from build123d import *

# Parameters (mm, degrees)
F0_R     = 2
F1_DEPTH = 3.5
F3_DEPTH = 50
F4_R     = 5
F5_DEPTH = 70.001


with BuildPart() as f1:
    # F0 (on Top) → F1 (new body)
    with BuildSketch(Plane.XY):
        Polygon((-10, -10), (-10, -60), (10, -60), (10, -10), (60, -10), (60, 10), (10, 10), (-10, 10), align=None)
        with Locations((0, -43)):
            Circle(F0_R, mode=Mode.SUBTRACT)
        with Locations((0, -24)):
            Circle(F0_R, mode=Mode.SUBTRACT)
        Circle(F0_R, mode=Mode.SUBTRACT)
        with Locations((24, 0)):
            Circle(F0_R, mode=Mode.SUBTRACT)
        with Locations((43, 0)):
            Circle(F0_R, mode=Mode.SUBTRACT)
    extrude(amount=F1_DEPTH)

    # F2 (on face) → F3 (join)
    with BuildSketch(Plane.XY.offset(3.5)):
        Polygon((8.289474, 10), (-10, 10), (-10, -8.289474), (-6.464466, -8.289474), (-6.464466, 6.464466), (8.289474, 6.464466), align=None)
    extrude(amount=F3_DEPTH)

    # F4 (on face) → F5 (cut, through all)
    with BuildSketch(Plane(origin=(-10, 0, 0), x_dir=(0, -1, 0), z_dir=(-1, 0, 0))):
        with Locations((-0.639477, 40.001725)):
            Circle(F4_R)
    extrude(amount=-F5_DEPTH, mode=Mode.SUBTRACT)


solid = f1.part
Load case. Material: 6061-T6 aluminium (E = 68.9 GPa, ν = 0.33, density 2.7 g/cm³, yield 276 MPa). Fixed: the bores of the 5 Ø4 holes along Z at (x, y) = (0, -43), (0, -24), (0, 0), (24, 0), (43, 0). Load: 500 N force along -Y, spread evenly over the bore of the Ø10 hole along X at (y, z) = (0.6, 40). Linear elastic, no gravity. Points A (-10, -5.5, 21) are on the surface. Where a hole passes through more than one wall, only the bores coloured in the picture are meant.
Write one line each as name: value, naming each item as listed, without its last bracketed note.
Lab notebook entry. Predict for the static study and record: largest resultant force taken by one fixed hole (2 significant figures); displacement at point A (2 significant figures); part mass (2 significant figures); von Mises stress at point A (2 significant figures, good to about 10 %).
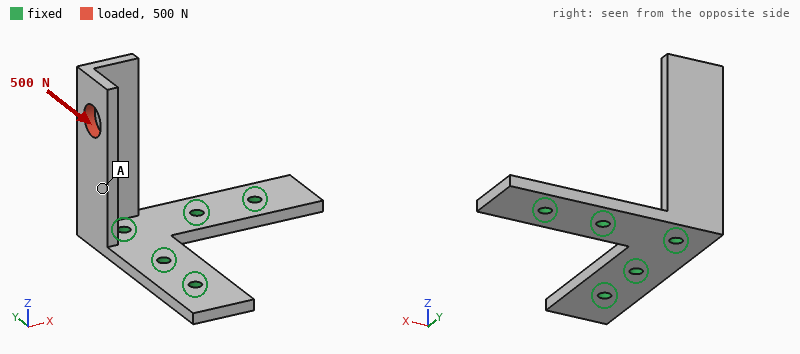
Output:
largest resultant force taken by one fixed hole: 570 N
displacement at point A: 0.19 mm
part mass: 37 g
von Mises stress at point A: 30 MPa
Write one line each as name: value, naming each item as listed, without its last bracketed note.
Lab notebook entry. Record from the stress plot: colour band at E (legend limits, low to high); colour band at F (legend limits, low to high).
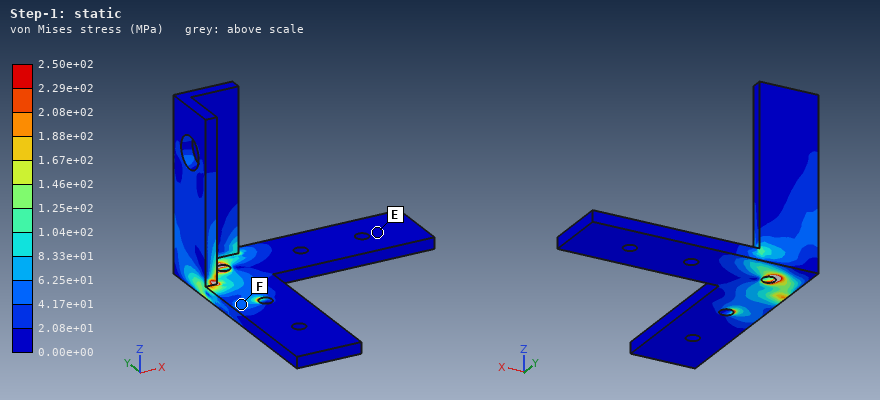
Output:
colour band at E: 0.00e+00 to 2.08e+01 MPa
colour band at F: 4.17e+01 to 6.25e+01 MPa
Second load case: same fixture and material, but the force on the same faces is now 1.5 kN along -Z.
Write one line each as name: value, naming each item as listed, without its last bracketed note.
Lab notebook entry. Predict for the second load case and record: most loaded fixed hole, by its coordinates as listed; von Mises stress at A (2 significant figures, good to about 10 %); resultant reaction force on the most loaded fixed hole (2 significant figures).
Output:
most loaded fixed hole, by its coordinates as listed: (0, 0)
von Mises stress at A: 27 MPa
resultant reaction force on the most loaded fixed hole: 1.6 kN
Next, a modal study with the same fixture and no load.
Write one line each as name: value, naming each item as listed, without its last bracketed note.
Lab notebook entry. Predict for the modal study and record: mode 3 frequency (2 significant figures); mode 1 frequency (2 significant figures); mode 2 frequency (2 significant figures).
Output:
mode 3 frequency: 5000 Hz
mode 1 frequency: 1500 Hz
mode 2 frequency: 2200 Hz
